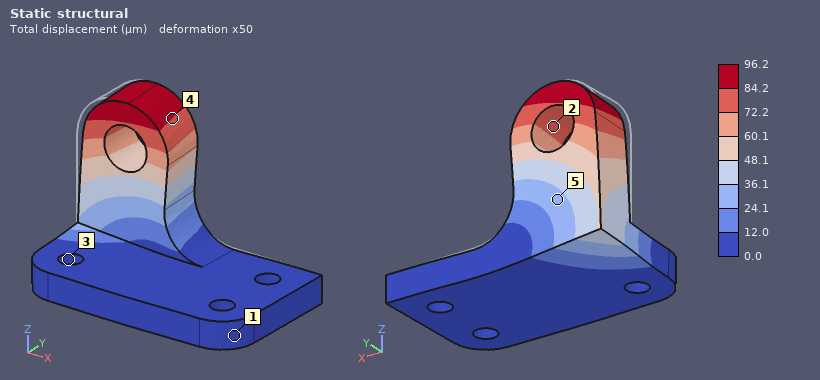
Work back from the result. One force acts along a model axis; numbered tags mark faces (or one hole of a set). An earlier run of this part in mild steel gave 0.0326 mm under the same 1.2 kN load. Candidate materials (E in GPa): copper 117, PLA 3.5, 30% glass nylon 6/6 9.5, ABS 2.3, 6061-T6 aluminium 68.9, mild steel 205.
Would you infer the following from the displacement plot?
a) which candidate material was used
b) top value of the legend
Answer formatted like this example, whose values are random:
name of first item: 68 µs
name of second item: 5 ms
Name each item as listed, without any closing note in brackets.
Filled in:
which candidate material was used: 6061-T6 aluminium
top value of the legend: 96.2 µm
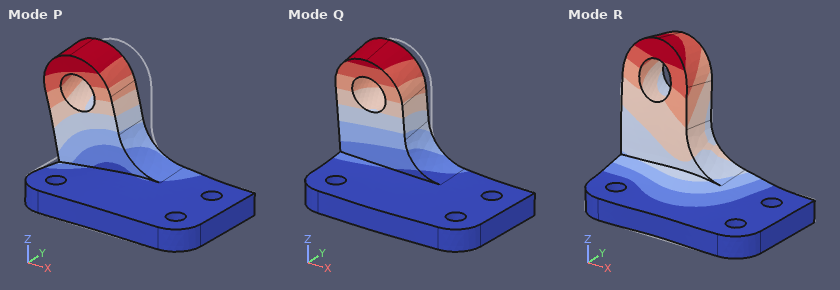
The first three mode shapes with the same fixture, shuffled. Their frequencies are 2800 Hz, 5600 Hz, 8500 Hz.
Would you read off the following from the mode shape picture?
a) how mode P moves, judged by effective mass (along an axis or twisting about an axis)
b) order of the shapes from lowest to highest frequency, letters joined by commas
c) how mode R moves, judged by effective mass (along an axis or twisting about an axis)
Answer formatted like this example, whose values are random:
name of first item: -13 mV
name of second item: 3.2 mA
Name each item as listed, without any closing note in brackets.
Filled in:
how mode P moves, judged by effective mass: along X
order of the shapes from lowest to highest frequency, letters joined by commas: Q, P, R
how mode R moves, judged by effective mass: along Z
